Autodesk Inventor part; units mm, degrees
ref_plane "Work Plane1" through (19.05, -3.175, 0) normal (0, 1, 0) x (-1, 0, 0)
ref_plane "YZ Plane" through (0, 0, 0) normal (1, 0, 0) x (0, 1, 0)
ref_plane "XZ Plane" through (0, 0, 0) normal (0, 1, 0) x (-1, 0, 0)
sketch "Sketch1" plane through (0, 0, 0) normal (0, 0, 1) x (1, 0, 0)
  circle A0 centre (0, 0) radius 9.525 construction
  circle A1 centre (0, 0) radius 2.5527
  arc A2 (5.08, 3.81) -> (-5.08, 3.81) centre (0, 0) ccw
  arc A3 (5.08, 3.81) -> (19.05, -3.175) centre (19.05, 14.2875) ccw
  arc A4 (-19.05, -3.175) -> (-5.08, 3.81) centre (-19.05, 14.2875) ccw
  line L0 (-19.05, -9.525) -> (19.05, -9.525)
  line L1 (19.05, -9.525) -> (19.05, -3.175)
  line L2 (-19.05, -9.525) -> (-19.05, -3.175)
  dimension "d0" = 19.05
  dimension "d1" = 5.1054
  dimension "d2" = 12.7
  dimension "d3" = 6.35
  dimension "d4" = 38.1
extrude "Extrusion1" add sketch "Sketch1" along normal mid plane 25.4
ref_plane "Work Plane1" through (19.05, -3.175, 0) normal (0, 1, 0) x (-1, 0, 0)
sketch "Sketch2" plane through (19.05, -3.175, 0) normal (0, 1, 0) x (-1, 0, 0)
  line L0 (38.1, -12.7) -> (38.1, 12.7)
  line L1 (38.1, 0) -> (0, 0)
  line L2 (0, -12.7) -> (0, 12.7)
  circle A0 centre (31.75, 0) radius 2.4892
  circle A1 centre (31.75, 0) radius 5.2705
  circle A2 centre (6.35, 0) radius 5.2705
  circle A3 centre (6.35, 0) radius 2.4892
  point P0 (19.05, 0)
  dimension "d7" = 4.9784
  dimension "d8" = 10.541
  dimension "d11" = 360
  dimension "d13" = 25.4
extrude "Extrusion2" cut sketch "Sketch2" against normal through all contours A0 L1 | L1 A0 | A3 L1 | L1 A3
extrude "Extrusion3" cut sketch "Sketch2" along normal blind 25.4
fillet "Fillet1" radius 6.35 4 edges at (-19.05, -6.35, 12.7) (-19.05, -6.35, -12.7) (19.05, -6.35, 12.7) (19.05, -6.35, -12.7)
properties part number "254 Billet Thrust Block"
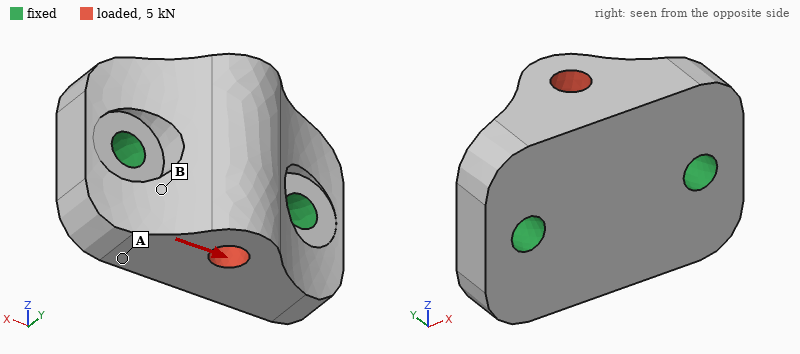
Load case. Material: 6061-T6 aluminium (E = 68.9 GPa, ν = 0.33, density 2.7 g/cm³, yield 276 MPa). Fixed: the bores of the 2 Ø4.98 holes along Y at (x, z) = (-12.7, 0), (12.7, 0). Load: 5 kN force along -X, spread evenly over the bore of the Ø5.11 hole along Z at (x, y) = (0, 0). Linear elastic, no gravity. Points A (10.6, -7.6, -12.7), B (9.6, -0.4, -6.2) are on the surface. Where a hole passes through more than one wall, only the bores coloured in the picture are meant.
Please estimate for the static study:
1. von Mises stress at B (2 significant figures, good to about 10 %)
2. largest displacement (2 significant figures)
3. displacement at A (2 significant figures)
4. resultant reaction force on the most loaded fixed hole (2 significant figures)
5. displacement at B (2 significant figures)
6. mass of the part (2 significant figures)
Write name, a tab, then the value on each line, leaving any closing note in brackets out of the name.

von Mises stress at B	28 MPa
largest displacement	8.6 µm
displacement at A	4.2 µm
resultant reaction force on the most loaded fixed hole	2.8 kN
displacement at B	5.1 µm
mass of the part	23 g
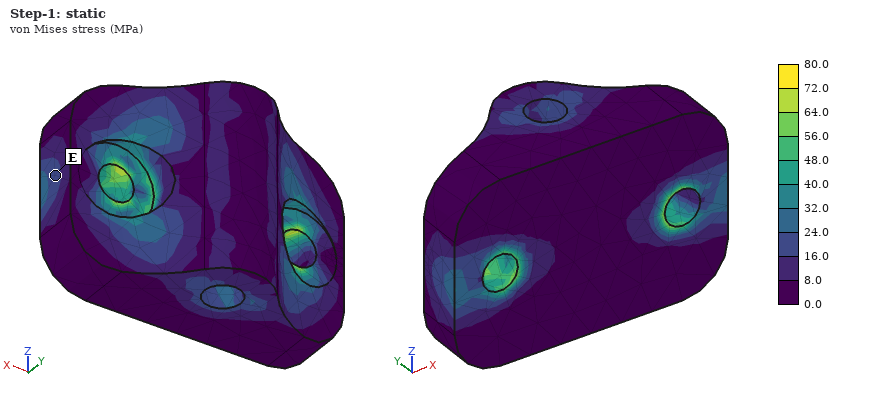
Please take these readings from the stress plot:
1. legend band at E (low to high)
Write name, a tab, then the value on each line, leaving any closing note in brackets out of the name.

legend band at E	16.0 to 24.0 MPa
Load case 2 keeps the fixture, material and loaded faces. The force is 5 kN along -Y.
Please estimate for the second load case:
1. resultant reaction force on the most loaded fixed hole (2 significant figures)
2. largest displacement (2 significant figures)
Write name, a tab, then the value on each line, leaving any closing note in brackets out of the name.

resultant reaction force on the most loaded fixed hole	2.7 kN
largest displacement	13 µm
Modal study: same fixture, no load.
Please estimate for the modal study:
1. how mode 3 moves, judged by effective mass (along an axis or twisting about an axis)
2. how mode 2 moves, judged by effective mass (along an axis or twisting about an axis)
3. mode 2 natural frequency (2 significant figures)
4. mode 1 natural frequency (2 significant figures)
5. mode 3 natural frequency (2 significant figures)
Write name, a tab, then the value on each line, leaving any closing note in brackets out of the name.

how mode 3 moves, judged by effective mass	along X
how mode 2 moves, judged by effective mass	along Y
mode 2 natural frequency	28 kHz
mode 1 natural frequency	17 kHz
mode 3 natural frequency	38 kHz
